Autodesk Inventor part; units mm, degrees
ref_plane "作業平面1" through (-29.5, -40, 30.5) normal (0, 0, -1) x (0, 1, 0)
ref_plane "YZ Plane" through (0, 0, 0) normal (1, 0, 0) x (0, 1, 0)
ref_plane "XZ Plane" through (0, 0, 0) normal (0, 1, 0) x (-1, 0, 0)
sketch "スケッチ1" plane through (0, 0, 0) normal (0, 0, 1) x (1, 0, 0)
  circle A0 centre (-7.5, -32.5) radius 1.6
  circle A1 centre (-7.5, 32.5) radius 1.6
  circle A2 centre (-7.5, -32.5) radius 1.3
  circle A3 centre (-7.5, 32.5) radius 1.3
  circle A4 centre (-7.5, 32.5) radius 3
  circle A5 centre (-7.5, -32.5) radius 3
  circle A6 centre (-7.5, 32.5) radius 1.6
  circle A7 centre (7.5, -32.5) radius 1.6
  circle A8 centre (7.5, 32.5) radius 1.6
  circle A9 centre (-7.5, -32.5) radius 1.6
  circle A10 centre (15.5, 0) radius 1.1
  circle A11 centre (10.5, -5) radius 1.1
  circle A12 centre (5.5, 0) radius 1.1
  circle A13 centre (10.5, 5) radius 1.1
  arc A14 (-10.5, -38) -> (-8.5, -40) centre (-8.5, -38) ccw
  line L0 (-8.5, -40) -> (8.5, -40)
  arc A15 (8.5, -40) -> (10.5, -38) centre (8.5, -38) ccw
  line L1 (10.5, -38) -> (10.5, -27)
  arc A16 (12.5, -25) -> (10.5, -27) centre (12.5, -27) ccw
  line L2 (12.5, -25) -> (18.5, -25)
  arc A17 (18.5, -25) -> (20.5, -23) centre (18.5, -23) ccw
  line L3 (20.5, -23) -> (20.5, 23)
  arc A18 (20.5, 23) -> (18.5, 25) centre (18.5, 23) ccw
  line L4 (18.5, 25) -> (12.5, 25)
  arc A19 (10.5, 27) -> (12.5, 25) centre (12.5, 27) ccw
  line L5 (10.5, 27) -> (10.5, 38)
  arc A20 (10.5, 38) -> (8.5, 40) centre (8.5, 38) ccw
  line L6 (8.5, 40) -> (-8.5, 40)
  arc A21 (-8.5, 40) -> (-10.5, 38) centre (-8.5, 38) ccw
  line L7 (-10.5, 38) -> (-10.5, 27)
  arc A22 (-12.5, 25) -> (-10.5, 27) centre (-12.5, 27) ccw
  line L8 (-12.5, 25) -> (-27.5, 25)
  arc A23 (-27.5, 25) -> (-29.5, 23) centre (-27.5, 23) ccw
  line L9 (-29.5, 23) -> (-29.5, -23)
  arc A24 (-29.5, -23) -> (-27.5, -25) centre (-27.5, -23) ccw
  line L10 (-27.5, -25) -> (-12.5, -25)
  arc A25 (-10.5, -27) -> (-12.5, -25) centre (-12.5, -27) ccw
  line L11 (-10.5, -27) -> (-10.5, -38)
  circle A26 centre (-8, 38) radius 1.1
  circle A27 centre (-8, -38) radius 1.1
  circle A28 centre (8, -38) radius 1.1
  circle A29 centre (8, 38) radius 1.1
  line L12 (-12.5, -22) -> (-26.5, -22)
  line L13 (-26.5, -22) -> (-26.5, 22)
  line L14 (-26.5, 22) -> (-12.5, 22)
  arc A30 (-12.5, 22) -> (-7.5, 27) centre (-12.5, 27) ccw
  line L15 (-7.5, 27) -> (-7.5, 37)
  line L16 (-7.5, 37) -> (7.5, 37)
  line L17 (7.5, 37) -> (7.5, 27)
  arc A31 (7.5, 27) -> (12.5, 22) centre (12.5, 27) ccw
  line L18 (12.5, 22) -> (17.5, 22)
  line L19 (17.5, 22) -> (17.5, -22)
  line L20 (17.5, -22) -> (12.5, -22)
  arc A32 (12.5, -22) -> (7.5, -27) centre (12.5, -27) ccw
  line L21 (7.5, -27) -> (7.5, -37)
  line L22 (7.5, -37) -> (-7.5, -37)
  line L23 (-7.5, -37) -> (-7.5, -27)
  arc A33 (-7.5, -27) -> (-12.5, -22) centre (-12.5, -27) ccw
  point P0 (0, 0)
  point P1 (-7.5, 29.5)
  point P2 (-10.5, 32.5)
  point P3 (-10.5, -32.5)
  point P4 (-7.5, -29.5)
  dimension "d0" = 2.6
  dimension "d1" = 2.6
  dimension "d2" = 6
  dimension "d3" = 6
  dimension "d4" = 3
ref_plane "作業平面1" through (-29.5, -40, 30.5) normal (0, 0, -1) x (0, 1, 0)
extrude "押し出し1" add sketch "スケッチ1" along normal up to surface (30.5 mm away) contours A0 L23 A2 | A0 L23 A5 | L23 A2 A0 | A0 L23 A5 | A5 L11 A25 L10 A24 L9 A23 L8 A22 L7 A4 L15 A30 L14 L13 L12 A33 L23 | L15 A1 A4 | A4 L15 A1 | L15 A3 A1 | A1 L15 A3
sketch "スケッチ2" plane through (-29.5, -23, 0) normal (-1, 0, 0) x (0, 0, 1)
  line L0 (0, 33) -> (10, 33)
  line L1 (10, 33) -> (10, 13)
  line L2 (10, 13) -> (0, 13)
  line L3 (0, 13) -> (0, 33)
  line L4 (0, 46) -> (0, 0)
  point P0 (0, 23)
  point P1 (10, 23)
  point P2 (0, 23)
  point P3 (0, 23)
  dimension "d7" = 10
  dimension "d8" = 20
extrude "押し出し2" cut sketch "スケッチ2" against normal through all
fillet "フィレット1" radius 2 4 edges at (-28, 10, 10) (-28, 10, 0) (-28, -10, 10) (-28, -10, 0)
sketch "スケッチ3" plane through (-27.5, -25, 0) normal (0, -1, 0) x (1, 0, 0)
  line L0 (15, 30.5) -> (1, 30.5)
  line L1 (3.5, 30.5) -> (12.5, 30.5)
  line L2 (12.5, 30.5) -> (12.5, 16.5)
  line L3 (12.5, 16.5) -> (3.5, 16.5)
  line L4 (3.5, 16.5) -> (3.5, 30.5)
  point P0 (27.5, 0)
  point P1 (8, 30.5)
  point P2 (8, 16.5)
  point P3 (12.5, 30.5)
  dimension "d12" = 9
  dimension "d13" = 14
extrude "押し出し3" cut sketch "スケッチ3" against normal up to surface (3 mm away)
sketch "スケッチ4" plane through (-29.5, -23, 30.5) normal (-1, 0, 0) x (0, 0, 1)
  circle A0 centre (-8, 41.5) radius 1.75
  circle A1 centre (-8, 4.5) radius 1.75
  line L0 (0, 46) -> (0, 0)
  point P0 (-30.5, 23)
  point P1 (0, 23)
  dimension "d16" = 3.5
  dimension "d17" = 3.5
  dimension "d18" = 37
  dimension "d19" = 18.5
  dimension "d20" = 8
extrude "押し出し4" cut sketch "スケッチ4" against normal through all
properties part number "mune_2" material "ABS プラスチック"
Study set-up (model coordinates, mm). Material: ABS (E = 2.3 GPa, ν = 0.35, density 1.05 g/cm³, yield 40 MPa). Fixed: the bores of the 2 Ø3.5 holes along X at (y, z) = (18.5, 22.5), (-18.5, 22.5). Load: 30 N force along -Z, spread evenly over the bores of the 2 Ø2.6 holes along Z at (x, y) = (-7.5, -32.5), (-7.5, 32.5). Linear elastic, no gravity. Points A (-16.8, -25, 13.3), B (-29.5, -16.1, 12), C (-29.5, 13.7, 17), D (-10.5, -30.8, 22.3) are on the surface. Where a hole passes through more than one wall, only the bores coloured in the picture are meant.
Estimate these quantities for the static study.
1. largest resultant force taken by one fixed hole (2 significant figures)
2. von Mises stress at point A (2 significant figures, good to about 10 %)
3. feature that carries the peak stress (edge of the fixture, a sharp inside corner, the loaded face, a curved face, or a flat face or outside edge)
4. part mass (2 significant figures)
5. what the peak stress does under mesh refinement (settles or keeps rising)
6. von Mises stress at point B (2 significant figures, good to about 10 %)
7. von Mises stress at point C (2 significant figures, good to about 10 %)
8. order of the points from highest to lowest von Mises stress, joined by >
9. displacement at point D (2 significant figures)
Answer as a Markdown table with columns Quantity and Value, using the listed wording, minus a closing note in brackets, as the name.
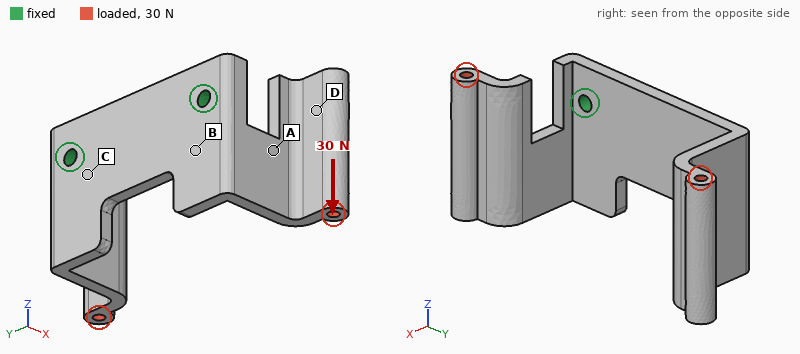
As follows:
| Quantity | Value |
|---|---|
| largest resultant force taken by one fixed hole | 16 N |
| von Mises stress at point A | 5.3 MPa |
| feature that carries the peak stress | edge of the fixture |
| part mass | 9.5 g |
| what the peak stress does under mesh refinement | keeps rising |
| von Mises stress at point B | 3.7 MPa |
| von Mises stress at point C | 2.1 MPa |
| order of the points from highest to lowest von Mises stress, joined by > | A > B > C > D |
| displacement at point D | 0.48 mm |
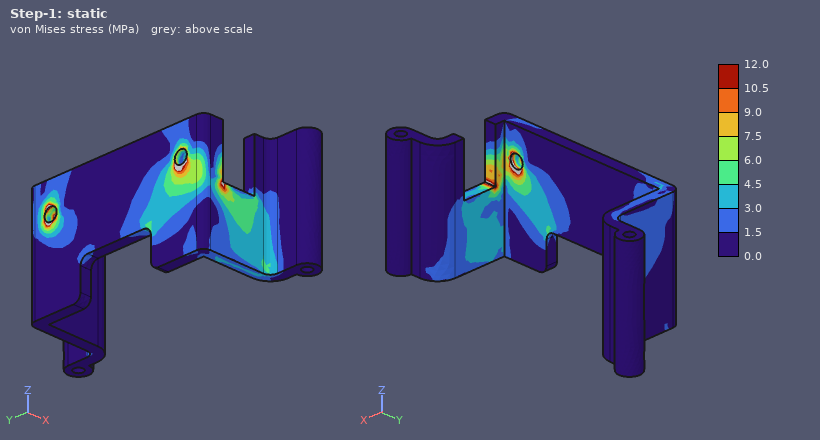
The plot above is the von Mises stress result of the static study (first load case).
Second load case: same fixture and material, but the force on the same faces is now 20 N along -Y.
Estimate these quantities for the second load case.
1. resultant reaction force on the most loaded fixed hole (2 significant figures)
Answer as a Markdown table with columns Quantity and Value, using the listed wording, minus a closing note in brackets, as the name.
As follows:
| Quantity | Value |
|---|---|
| resultant reaction force on the most loaded fixed hole | 12 N |
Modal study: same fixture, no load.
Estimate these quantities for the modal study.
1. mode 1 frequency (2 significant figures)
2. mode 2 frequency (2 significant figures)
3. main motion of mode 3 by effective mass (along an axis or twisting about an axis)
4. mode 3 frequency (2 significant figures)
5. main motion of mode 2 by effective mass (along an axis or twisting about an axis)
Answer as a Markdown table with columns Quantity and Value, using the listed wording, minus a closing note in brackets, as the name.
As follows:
| Quantity | Value |
|---|---|
| mode 1 frequency | 450 Hz |
| mode 2 frequency | 610 Hz |
| main motion of mode 3 by effective mass | along Z |
| mode 3 frequency | 660 Hz |
| main motion of mode 2 by effective mass | along Y |
